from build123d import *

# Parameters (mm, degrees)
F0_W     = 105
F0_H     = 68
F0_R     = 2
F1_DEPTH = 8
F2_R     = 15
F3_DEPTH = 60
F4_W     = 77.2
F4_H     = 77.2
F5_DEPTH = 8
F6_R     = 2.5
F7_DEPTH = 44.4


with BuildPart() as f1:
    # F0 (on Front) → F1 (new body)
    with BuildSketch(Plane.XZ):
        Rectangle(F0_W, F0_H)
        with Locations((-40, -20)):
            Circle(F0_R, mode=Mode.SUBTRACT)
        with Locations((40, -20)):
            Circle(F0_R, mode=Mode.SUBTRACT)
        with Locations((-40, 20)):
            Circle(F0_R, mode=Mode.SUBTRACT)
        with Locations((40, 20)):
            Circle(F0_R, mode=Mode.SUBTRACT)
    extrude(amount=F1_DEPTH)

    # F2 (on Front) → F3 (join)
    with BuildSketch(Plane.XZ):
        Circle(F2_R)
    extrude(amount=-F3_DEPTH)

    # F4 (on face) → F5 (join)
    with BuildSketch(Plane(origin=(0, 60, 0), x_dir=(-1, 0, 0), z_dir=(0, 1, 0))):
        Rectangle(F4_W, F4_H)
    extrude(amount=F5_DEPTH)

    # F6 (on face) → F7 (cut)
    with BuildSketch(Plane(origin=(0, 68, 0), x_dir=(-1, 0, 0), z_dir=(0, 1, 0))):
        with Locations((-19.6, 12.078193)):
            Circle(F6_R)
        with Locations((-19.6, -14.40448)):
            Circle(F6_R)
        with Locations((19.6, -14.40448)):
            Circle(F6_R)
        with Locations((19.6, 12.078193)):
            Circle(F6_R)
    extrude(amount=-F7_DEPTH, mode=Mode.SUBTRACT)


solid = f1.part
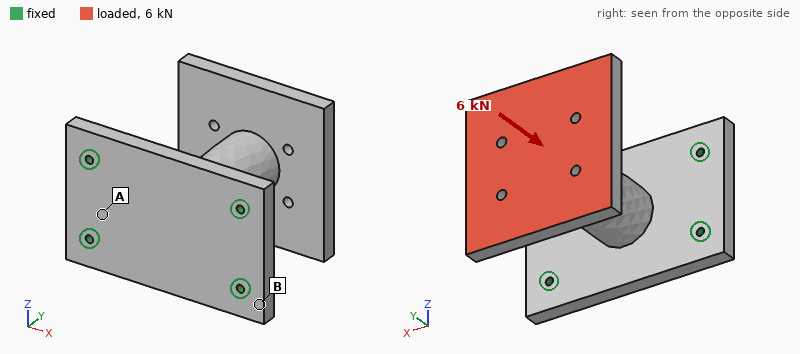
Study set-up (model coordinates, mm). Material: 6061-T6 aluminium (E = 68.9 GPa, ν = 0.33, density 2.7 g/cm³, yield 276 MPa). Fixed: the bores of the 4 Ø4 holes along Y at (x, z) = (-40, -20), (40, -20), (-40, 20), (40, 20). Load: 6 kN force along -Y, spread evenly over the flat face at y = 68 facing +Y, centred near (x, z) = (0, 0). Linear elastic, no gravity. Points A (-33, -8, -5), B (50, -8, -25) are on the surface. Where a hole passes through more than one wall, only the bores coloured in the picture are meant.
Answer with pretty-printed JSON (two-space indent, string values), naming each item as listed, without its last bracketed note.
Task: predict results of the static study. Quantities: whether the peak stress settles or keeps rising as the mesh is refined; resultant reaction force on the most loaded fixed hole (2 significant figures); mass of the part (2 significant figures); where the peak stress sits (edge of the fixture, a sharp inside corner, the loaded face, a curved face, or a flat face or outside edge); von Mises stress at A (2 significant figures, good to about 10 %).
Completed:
{
  "whether the peak stress settles or keeps rising as the mesh is refined": "keeps rising",
  "resultant reaction force on the most loaded fixed hole": "1.6 kN",
  "mass of the part": "390 g",
  "where the peak stress sits": "edge of the fixture",
  "von Mises stress at A": "23 MPa"
}
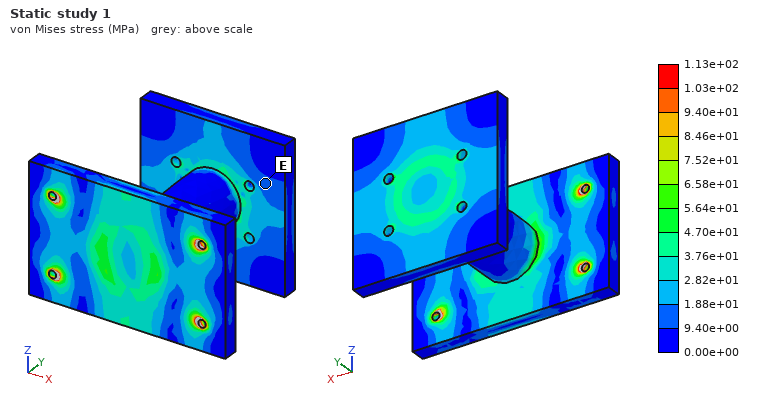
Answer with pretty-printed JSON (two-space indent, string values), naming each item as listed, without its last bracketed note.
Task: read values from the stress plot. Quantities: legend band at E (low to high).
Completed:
{
  "legend band at E": "9.40e+00 to 1.88e+01 MPa"
}
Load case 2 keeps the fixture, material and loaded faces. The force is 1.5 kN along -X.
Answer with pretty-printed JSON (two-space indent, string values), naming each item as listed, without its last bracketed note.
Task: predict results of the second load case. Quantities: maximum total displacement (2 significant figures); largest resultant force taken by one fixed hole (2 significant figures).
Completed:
{
  "maximum total displacement": "0.22 mm",
  "largest resultant force taken by one fixed hole": "950 N"
}
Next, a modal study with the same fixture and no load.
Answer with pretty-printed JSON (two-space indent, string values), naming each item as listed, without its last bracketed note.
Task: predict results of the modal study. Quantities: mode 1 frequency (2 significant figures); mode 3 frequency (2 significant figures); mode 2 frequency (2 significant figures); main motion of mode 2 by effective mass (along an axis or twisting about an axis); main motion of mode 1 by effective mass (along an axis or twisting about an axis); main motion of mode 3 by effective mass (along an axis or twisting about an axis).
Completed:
{
  "mode 1 frequency": "910 Hz",
  "mode 3 frequency": "2400 Hz",
  "mode 2 frequency": "1200 Hz",
  "main motion of mode 2 by effective mass": "along X",
  "main motion of mode 1 by effective mass": "along Z",
  "main motion of mode 3 by effective mass": "twisting about Y"
}
